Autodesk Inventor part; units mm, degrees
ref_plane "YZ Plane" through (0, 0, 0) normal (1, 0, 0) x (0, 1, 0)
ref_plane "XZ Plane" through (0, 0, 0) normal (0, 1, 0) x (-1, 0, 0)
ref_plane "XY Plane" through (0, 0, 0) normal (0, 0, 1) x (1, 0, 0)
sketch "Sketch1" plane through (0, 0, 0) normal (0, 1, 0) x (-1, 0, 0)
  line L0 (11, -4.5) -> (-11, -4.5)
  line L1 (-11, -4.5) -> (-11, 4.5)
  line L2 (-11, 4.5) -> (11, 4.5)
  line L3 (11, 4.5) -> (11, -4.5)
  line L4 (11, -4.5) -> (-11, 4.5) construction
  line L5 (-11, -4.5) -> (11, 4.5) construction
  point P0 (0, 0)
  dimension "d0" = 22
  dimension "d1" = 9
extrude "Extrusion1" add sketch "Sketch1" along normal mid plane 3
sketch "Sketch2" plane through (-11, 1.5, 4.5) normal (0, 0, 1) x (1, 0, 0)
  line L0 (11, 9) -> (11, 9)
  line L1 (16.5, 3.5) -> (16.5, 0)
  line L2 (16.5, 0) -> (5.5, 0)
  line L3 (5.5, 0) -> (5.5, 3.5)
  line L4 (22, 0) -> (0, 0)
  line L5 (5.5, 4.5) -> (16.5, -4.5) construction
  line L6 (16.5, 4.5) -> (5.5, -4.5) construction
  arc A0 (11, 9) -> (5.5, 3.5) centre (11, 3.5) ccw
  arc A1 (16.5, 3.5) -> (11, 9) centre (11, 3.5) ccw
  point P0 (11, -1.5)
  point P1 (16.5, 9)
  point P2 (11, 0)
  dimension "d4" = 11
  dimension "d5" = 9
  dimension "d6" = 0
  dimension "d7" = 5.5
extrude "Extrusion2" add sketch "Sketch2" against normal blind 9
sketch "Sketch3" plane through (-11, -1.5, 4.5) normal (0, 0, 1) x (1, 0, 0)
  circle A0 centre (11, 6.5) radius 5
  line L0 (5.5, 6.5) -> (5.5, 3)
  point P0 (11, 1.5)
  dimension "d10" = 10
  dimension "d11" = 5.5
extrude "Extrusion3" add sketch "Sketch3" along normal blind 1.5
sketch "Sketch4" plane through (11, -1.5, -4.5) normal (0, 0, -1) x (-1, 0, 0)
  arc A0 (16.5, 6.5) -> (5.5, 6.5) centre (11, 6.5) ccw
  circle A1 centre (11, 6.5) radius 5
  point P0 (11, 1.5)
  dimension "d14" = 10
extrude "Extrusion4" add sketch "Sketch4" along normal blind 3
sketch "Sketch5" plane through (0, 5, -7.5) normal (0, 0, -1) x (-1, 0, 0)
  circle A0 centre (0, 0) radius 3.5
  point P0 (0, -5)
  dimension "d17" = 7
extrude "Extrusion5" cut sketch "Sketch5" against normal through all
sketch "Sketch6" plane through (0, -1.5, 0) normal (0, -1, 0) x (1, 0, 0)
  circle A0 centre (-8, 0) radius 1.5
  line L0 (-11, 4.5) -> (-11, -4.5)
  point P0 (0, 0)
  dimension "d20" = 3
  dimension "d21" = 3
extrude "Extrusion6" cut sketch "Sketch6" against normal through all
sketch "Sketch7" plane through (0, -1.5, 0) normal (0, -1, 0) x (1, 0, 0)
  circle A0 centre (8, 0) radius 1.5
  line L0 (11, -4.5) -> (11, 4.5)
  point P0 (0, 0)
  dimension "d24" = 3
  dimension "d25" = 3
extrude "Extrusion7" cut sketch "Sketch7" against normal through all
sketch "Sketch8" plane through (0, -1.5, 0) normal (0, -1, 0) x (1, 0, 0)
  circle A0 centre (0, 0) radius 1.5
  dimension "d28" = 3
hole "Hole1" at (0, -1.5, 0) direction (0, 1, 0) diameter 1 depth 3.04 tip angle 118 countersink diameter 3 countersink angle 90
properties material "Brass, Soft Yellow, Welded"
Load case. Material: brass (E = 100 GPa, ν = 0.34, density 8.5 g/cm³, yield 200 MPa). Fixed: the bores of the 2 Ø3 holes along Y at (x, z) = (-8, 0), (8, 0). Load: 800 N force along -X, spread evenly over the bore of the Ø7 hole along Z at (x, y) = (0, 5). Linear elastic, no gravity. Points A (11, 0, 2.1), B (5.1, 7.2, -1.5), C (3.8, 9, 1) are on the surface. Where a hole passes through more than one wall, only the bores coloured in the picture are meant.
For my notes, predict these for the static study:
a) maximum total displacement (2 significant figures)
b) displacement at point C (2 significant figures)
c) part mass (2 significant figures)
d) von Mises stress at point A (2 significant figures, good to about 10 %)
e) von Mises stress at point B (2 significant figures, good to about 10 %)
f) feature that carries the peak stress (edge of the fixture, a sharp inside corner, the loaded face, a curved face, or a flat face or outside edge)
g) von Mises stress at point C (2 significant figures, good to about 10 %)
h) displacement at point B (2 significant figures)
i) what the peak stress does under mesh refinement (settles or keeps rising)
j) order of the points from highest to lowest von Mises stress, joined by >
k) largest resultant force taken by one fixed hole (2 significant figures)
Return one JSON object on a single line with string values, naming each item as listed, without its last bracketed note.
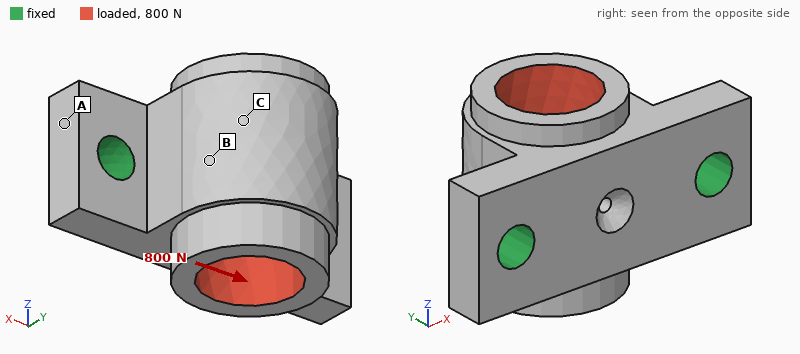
{"maximum total displacement": "9.8 µm", "displacement at point C": "8.9 µm", "part mass": "9.8 g", "von Mises stress at point A": "5.2 MPa", "von Mises stress at point B": "18 MPa", "feature that carries the peak stress": "a sharp inside corner", "von Mises stress at point C": "23 MPa", "displacement at point B": "8.0 µm", "what the peak stress does under mesh refinement": "keeps rising", "order of the points from highest to lowest von Mises stress, joined by >": "C > B > A", "largest resultant force taken by one fixed hole": "500 N"}
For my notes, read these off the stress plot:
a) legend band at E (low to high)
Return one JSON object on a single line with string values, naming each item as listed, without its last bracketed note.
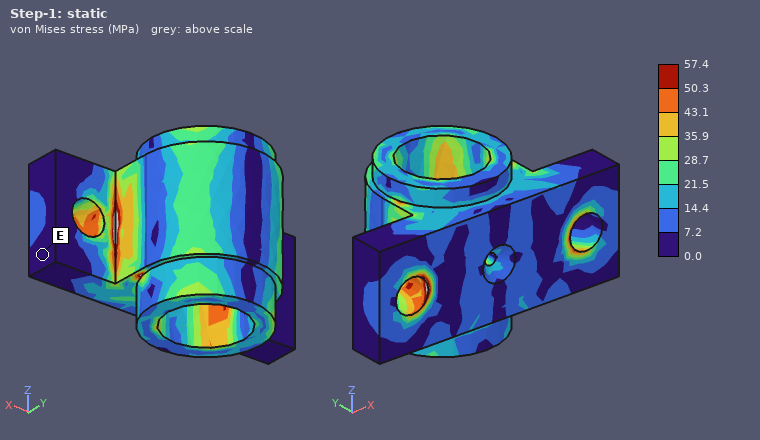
{"legend band at E": "0.0 to 7.2 MPa"}
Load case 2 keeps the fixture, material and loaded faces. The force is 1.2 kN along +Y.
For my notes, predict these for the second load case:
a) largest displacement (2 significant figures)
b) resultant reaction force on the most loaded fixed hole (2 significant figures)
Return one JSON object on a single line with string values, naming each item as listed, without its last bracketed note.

{"largest displacement": "10 µm", "resultant reaction force on the most loaded fixed hole": "620 N"}
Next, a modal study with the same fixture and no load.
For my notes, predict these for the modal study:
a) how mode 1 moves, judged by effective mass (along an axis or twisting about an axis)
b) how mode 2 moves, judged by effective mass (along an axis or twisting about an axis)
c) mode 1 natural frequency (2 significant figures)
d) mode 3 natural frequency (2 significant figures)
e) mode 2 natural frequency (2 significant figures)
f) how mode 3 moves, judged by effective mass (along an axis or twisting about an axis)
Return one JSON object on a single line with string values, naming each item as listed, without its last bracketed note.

{"how mode 1 moves, judged by effective mass": "along Z", "how mode 2 moves, judged by effective mass": "along X", "mode 1 natural frequency": "13 kHz", "mode 3 natural frequency": "30 kHz", "mode 2 natural frequency": "21 kHz", "how mode 3 moves, judged by effective mass": "along Y"}
